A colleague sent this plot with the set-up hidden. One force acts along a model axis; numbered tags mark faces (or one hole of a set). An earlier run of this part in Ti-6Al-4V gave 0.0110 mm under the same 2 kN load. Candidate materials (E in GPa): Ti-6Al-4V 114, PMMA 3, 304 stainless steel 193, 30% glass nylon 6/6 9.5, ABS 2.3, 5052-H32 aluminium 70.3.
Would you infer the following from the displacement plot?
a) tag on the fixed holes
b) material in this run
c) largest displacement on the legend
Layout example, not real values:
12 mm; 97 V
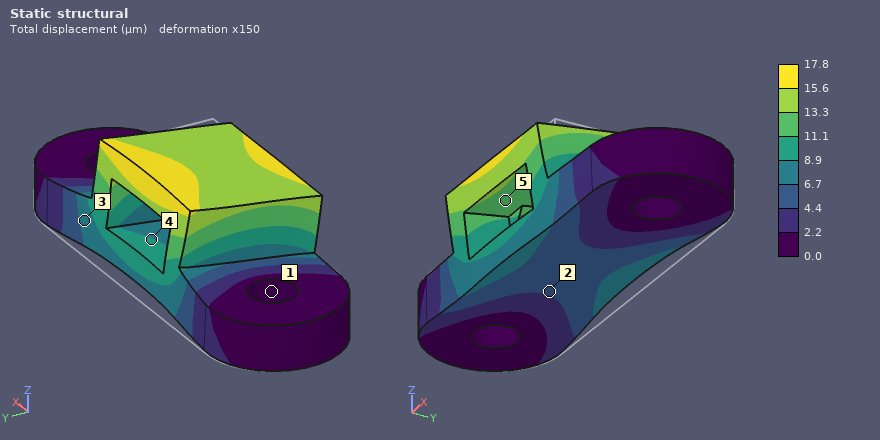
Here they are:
1; 5052-H32 aluminium; 17.8 µm
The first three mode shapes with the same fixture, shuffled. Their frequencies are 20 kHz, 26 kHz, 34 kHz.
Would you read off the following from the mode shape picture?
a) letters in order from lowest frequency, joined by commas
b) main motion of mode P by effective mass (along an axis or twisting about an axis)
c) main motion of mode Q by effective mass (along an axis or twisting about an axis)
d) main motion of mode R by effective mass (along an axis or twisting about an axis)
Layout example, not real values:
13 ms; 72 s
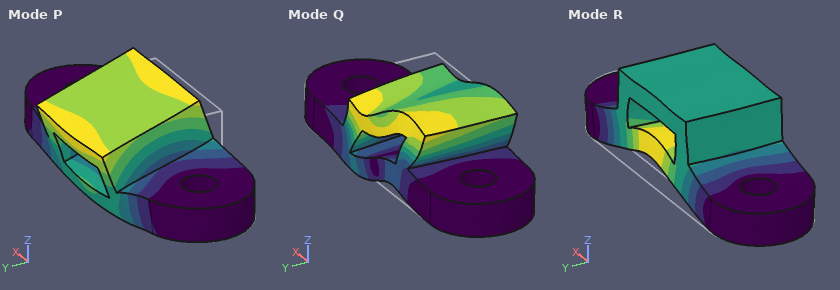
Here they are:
P, R, Q; along Y; along X; along Z
